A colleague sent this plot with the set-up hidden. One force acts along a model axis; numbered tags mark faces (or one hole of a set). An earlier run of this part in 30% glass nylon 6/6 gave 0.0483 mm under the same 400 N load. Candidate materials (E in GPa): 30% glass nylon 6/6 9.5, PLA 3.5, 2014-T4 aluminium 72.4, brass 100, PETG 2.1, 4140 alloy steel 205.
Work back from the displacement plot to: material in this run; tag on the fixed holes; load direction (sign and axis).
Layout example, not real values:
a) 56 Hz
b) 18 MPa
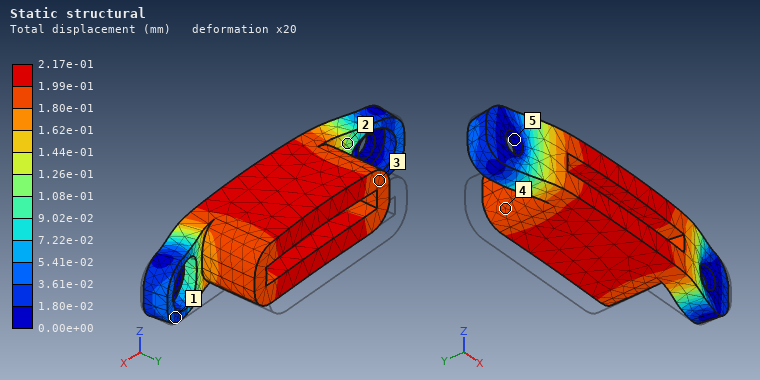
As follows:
a) PETG
b) 5
c) -Y
